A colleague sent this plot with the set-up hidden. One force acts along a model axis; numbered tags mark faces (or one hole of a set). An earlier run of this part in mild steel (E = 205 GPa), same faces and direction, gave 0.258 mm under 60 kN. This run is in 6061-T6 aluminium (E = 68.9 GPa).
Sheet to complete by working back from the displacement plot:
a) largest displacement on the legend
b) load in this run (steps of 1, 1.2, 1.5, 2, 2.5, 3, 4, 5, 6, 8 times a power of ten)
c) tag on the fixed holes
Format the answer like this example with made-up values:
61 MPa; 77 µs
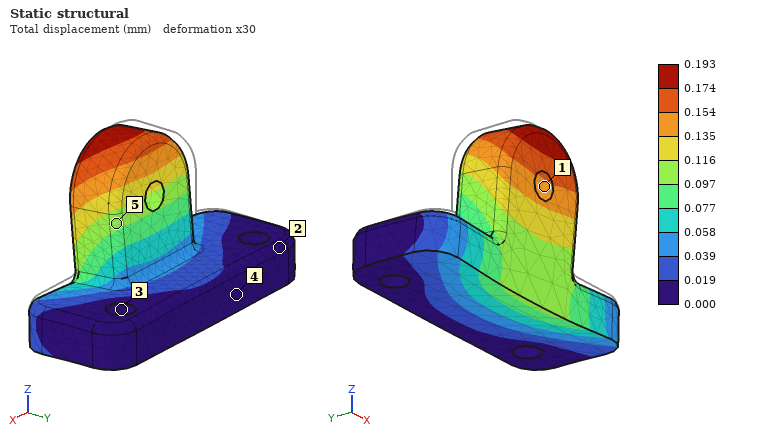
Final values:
0.193 mm; 15 kN; 3
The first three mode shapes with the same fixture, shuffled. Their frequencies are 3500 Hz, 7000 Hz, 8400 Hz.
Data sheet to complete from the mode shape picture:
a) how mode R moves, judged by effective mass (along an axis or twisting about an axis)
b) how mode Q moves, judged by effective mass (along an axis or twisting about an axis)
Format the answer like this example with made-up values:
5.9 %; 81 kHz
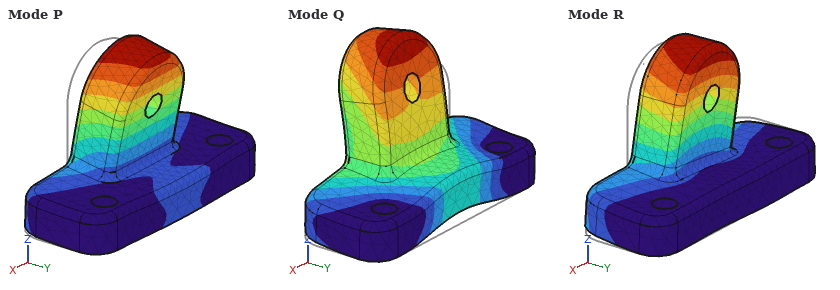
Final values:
along X; along Z
